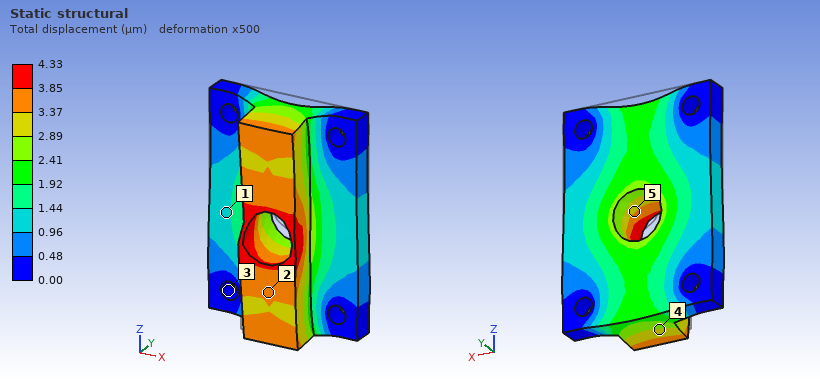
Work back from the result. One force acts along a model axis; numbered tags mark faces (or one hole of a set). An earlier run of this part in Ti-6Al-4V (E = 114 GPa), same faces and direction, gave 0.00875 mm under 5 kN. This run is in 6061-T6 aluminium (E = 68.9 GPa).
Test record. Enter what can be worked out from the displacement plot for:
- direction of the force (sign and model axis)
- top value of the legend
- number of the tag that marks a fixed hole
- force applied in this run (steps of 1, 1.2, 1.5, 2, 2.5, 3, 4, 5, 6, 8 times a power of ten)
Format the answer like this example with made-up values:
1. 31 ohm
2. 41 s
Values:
1. -Z
2. 4.33 µm
3. 3
4. 1.5 kN
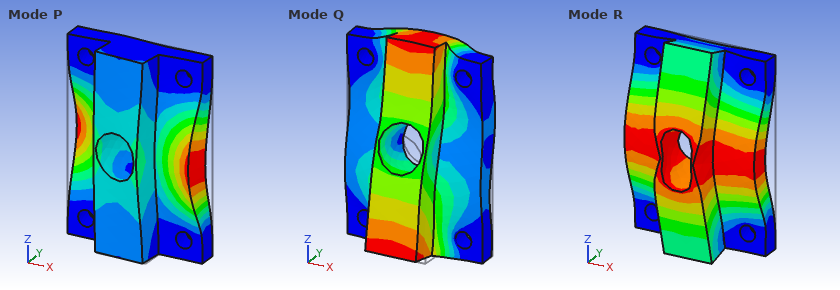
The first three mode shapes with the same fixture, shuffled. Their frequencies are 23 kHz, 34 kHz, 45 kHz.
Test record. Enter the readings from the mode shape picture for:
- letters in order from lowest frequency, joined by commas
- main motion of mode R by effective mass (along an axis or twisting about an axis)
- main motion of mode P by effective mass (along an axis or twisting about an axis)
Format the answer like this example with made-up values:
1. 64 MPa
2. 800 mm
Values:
1. R, P, Q
2. along Y
3. twisting about Z
